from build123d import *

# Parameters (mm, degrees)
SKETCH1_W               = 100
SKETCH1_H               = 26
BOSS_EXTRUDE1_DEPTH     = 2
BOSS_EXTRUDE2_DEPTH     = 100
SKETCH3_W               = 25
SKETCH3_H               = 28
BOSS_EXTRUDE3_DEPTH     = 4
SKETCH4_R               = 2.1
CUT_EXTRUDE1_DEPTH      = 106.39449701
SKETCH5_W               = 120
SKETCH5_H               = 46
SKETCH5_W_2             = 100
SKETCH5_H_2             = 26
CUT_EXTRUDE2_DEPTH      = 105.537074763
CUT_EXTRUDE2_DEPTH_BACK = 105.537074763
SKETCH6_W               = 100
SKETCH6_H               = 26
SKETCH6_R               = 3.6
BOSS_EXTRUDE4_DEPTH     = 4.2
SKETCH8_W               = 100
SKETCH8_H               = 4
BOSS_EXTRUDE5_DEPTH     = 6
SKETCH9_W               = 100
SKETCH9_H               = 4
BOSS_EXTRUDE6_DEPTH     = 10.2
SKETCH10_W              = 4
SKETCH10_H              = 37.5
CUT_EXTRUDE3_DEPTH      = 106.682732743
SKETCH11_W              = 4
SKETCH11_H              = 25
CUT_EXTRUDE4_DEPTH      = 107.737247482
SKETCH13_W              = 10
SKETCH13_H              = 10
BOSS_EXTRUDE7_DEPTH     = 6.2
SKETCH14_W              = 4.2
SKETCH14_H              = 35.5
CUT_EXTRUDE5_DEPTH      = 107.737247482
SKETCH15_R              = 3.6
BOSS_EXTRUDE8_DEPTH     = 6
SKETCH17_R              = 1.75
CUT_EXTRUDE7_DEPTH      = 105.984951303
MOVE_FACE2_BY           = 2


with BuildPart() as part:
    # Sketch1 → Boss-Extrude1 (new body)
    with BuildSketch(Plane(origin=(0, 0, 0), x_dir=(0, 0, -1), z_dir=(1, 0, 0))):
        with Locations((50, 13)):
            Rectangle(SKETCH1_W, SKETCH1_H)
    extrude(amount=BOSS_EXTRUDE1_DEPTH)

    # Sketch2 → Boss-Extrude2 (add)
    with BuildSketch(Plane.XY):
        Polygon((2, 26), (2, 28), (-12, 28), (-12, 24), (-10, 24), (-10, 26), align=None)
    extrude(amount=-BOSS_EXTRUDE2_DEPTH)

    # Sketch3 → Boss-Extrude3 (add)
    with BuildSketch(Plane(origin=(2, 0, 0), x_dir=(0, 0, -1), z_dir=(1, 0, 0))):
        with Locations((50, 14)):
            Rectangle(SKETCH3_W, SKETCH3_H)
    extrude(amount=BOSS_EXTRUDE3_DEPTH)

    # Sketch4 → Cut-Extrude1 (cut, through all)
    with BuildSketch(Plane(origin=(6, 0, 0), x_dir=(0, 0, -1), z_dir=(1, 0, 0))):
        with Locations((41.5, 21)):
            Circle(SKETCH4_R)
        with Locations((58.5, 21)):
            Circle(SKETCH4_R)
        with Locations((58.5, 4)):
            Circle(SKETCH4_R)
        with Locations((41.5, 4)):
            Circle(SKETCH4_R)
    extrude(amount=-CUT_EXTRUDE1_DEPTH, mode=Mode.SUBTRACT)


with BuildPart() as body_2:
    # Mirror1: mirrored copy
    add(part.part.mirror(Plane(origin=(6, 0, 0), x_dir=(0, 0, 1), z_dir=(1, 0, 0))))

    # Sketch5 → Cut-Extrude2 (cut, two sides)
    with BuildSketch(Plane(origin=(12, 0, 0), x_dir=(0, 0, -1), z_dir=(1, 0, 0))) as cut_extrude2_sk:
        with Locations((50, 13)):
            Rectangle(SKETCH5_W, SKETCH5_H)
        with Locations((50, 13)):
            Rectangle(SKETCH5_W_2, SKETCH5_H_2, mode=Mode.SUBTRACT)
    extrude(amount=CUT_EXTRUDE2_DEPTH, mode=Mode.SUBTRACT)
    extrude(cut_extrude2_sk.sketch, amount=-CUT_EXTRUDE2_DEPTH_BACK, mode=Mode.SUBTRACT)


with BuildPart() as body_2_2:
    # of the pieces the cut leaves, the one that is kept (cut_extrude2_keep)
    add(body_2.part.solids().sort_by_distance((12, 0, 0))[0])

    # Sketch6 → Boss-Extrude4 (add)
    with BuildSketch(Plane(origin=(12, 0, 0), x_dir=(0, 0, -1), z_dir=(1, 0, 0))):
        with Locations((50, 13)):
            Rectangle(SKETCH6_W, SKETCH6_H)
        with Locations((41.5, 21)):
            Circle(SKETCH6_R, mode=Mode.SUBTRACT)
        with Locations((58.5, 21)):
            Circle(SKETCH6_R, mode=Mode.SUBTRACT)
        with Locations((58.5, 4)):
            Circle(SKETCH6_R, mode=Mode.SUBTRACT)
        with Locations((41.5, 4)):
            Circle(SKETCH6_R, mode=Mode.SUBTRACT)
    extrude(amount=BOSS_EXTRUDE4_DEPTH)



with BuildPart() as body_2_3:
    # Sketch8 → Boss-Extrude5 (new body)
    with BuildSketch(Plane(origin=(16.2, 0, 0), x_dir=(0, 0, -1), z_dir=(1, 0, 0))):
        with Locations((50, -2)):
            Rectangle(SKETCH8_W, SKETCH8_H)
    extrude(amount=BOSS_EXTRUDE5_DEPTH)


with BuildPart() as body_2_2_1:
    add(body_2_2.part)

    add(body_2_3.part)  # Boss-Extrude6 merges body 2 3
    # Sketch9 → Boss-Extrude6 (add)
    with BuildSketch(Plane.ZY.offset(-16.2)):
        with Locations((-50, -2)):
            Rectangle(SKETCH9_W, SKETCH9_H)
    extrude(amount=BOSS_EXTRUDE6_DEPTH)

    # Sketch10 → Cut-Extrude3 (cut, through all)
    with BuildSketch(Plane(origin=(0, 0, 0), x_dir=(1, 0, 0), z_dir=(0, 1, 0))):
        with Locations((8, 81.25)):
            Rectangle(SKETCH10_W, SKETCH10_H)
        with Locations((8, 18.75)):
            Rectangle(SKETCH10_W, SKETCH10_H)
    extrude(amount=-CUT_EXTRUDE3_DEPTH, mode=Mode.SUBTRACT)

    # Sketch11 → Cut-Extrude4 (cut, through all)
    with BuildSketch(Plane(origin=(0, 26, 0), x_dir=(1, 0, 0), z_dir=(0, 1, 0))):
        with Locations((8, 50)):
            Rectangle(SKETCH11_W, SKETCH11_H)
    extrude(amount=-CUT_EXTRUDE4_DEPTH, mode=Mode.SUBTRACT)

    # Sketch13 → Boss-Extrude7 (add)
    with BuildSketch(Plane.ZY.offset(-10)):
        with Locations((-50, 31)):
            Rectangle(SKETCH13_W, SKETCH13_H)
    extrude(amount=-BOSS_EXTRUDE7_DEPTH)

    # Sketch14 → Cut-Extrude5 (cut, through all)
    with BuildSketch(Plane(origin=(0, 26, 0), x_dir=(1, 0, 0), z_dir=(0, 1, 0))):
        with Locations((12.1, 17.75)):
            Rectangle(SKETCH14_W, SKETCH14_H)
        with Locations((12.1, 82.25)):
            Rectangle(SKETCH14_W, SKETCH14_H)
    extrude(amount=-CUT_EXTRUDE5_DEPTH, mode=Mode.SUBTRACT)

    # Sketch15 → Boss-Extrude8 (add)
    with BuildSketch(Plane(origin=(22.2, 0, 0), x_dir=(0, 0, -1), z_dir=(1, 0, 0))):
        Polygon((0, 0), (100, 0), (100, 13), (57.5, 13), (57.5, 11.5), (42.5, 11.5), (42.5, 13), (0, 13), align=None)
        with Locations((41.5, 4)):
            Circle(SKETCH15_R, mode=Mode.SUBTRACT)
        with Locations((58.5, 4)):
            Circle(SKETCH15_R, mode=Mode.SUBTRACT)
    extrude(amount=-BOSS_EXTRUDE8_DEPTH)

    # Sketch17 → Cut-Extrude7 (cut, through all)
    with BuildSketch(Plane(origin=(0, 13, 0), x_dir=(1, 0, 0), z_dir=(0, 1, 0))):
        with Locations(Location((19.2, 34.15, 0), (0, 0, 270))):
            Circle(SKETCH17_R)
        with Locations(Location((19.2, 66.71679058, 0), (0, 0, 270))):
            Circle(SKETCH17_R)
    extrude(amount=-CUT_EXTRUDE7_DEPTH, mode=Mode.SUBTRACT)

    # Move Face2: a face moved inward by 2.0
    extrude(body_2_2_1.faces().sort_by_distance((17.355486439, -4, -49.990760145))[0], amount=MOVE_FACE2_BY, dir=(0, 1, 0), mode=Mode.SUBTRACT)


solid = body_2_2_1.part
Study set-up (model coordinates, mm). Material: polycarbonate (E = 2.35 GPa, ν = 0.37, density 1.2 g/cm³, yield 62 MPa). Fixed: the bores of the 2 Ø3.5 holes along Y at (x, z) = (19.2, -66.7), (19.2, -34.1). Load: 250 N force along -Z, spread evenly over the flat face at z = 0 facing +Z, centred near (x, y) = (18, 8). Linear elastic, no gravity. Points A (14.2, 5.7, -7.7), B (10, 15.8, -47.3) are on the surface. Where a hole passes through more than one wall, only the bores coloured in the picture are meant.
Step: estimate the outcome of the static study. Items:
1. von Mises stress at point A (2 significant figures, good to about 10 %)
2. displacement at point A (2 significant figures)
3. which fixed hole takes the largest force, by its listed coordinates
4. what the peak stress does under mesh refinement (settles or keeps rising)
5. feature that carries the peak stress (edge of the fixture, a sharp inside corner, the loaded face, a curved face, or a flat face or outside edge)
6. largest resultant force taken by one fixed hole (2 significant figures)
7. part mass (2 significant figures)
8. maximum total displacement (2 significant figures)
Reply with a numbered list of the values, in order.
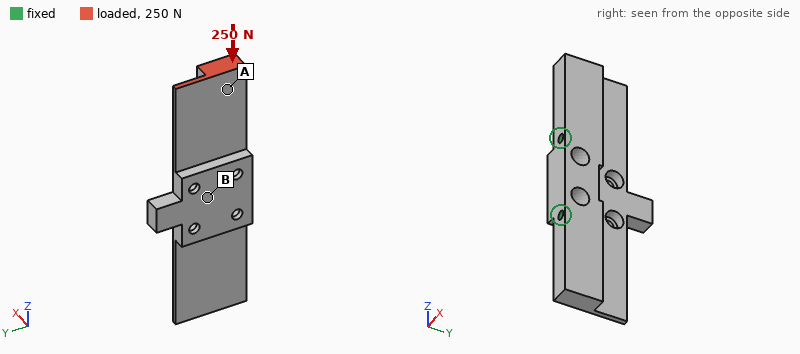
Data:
1. 1.7 MPa
2. 31 µm
3. (19.2, -34.1)
4. keeps rising
5. edge of the fixture
6. 230 N
7. 20 g
8. 45 µm
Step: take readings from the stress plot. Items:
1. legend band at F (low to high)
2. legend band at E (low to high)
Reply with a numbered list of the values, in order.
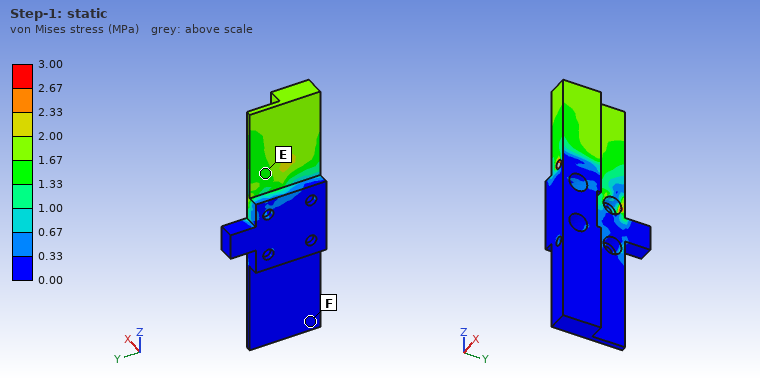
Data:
1. 0.00 to 0.33 MPa
2. 1.33 to 1.67 MPa
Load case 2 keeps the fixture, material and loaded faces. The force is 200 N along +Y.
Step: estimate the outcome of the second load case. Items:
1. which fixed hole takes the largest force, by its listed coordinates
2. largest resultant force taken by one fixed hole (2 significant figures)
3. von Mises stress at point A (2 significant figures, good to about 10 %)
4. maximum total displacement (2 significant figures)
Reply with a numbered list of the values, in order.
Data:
1. (19.2, -34.1)
2. 260 N
3. 3.4 MPa
4. 0.40 mm
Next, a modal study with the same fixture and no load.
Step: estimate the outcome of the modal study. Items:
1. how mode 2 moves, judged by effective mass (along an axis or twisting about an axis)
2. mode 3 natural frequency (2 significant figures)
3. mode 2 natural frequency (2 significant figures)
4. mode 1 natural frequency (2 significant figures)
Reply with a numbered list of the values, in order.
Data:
1. along X
2. 2200 Hz
3. 1400 Hz
4. 1300 Hz
